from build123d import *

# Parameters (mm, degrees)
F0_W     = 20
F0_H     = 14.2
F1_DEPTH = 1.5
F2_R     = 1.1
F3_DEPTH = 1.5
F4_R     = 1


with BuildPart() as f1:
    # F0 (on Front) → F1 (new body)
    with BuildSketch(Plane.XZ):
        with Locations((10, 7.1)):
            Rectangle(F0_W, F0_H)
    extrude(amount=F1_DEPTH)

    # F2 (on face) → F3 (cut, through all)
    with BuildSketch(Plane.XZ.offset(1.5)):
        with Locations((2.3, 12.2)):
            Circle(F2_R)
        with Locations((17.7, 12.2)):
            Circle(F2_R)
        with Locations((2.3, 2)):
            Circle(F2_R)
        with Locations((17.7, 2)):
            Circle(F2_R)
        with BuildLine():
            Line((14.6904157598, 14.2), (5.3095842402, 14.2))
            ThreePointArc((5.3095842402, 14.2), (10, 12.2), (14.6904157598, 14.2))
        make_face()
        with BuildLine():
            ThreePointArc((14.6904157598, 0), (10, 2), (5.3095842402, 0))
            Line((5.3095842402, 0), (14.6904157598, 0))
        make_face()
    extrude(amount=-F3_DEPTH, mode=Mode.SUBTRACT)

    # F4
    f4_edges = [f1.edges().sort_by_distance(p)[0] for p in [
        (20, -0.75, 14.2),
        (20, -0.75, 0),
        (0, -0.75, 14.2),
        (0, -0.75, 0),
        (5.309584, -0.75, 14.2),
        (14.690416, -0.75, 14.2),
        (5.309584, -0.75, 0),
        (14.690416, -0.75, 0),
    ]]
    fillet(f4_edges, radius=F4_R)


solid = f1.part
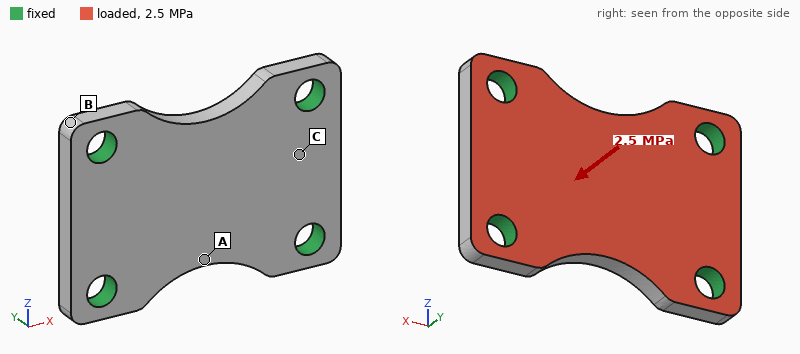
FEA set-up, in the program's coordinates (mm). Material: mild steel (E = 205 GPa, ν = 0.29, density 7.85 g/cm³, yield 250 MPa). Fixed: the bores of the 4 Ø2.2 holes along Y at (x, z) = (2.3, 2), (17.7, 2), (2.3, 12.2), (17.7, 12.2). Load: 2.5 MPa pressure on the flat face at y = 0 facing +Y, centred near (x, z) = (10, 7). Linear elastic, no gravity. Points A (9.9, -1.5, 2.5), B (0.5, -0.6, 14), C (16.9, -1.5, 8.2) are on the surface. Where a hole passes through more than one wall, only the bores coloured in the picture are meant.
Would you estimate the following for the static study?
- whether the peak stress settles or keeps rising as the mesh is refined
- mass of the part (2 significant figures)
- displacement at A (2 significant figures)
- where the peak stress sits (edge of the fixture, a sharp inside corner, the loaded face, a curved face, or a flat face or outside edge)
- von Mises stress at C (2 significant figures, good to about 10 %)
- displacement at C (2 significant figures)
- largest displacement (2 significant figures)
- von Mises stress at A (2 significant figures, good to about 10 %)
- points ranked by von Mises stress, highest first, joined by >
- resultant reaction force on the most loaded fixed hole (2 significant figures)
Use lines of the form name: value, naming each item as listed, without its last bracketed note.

whether the peak stress settles or keeps rising as the mesh is refined: keeps rising
mass of the part: 2.8 g
displacement at A: 5.5 µm
where the peak stress sits: edge of the fixture
von Mises stress at C: 36 MPa
displacement at C: 1.7 µm
largest displacement: 6.4 µm
von Mises stress at A: 67 MPa
points ranked by von Mises stress, highest first, joined by >: A > C > B
resultant reaction force on the most loaded fixed hole: 150 N
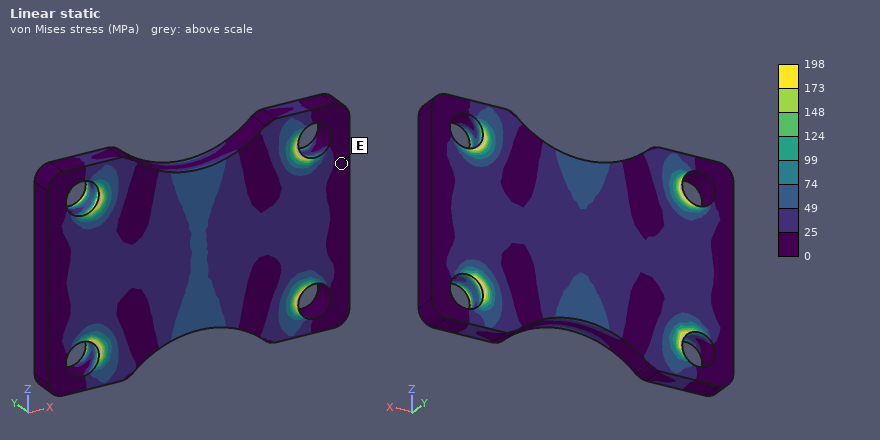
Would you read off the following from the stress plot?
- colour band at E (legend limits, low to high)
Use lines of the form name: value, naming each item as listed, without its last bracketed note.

colour band at E: 0 to 25 MPa
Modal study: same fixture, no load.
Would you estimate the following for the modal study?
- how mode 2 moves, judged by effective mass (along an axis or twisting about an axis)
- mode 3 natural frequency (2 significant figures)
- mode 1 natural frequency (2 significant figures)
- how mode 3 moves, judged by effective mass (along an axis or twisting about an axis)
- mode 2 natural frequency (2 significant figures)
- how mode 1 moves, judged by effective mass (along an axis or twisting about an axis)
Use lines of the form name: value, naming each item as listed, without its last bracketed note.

how mode 2 moves, judged by effective mass: twisting about X
mode 3 natural frequency: 75 kHz
mode 1 natural frequency: 34 kHz
how mode 3 moves, judged by effective mass: twisting about Z
mode 2 natural frequency: 55 kHz
how mode 1 moves, judged by effective mass: along Y
